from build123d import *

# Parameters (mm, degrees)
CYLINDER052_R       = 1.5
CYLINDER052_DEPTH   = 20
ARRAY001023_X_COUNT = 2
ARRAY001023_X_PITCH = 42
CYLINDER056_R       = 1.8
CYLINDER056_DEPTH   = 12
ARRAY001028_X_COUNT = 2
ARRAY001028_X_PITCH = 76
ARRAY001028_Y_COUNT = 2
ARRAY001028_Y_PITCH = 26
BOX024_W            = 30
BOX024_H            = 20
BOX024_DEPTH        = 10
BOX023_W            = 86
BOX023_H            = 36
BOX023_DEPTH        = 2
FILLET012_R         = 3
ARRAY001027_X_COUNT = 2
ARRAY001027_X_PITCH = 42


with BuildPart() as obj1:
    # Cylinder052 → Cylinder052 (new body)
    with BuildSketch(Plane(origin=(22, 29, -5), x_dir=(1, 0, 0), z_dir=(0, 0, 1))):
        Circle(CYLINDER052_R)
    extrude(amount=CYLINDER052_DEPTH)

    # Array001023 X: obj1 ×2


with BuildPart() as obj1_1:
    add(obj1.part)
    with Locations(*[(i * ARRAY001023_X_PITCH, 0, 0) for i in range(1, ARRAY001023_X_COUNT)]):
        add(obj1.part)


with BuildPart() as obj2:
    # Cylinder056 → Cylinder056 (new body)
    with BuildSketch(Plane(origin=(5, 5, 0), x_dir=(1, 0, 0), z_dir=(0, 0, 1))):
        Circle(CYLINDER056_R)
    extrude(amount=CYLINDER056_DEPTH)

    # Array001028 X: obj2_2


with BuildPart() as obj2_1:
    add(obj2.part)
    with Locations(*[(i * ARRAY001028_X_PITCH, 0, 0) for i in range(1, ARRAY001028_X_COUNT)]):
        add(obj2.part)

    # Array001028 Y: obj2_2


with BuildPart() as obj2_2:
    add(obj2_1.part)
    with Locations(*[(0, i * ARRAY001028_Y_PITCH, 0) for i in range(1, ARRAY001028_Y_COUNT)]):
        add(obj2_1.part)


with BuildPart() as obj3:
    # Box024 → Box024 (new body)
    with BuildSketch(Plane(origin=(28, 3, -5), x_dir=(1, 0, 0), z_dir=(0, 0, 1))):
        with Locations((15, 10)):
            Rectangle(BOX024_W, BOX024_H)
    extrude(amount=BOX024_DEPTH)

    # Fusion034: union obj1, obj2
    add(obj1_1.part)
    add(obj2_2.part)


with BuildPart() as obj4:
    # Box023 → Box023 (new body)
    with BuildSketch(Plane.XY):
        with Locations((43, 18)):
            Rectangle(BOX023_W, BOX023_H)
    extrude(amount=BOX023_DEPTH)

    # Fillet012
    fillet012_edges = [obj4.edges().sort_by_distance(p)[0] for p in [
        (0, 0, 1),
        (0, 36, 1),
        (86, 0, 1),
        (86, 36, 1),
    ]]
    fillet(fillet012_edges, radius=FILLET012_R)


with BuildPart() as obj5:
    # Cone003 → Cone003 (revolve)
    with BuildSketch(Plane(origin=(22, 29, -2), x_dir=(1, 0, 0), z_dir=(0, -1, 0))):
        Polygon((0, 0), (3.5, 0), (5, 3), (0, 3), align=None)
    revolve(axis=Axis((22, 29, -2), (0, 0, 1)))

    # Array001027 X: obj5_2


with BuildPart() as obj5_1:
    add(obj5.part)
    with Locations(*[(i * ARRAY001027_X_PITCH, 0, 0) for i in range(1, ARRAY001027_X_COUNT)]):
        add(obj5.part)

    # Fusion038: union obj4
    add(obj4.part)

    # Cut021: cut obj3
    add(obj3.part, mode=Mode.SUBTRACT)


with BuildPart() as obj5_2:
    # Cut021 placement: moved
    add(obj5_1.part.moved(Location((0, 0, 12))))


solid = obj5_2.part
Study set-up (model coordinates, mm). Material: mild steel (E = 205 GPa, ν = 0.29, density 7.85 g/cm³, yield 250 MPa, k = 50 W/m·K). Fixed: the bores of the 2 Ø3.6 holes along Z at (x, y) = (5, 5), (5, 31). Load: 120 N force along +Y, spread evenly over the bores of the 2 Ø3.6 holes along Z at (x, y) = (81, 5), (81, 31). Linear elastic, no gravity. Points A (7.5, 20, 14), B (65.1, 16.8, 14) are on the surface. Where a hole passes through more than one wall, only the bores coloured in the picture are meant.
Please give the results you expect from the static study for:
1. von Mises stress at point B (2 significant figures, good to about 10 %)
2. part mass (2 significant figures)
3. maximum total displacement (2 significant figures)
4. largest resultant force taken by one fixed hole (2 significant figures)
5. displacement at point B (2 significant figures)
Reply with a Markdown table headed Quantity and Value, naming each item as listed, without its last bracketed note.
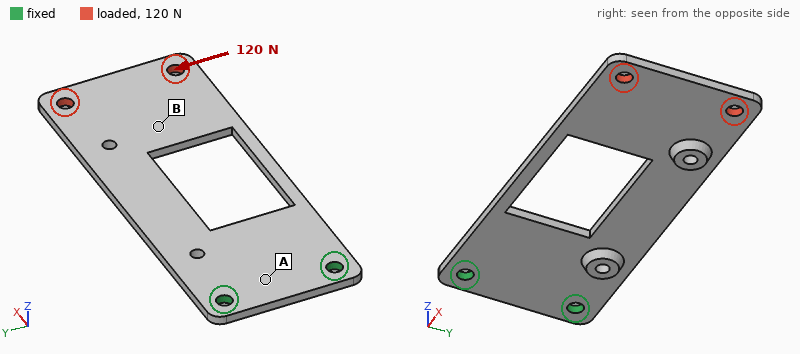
| Quantity | Value |
|---|---|
| von Mises stress at point B | 7.8 MPa |
| part mass | 40 g |
| maximum total displacement | 32 µm |
| largest resultant force taken by one fixed hole | 350 N |
| displacement at point B | 23 µm |
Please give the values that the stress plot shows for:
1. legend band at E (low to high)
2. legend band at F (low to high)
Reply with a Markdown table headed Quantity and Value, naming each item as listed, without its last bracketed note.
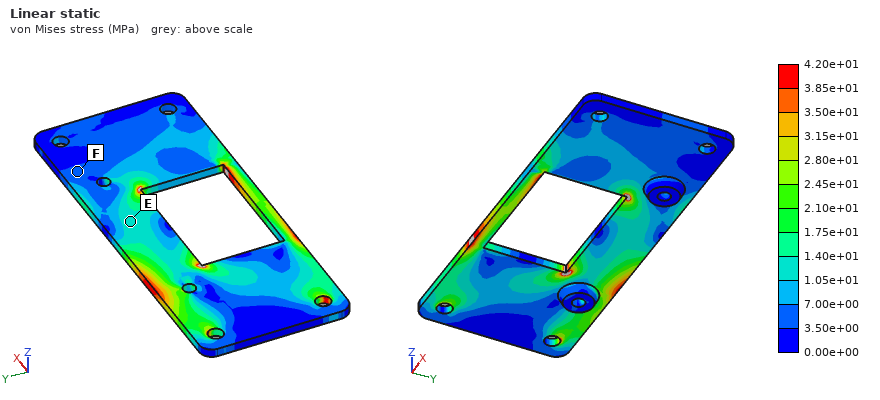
| Quantity | Value |
|---|---|
| legend band at E | 1.05e+01 to 1.40e+01 MPa |
| legend band at F | 3.50e+00 to 7.00e+00 MPa |
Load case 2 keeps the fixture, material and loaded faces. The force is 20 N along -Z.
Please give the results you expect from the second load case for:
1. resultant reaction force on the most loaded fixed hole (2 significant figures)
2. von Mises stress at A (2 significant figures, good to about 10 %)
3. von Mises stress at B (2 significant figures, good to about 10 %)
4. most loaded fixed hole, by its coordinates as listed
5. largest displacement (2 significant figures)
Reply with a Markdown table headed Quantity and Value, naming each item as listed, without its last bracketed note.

| Quantity | Value |
|---|---|
| resultant reaction force on the most loaded fixed hole | 12 N |
| von Mises stress at A | 34 MPa |
| von Mises stress at B | 10 MPa |
| most loaded fixed hole, by its coordinates as listed | (5, 5) |
| largest displacement | 0.96 mm |
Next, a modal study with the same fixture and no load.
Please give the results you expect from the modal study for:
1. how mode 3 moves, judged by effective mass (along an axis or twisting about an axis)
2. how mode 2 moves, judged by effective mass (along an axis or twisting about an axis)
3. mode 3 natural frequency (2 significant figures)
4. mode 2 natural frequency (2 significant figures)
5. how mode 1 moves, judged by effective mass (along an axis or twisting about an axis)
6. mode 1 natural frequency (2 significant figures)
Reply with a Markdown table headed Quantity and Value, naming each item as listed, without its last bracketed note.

| Quantity | Value |
|---|---|
| how mode 3 moves, judged by effective mass | along Z |
| how mode 2 moves, judged by effective mass | twisting about X |
| mode 3 natural frequency | 1600 Hz |
| mode 2 natural frequency | 1000 Hz |
| how mode 1 moves, judged by effective mass | along Z |
| mode 1 natural frequency | 230 Hz |
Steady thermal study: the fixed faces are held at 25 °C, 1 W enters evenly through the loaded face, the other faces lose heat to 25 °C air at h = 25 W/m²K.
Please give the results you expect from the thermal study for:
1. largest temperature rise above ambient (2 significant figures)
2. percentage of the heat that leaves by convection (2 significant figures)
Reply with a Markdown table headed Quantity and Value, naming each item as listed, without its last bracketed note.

| Quantity | Value |
|---|---|
| largest temperature rise above ambient | 14 K |
| percentage of the heat that leaves by convection | 78 % |
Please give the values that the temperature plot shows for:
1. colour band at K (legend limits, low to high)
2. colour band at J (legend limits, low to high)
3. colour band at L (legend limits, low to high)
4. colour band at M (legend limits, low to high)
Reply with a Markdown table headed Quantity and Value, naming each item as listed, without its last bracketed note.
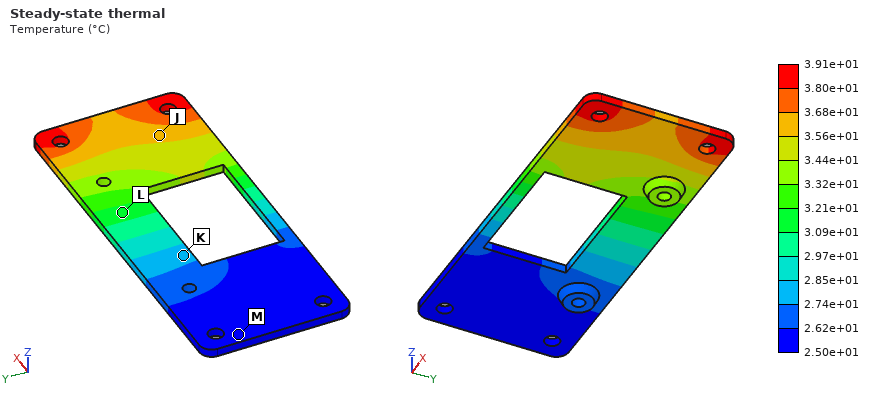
| Quantity | Value |
|---|---|
| colour band at K | 2.74e+01 to 2.85e+01 °C |
| colour band at J | 3.56e+01 to 3.68e+01 °C |
| colour band at L | 3.09e+01 to 3.21e+01 °C |
| colour band at M | 2.50e+01 to 2.62e+01 °C |
